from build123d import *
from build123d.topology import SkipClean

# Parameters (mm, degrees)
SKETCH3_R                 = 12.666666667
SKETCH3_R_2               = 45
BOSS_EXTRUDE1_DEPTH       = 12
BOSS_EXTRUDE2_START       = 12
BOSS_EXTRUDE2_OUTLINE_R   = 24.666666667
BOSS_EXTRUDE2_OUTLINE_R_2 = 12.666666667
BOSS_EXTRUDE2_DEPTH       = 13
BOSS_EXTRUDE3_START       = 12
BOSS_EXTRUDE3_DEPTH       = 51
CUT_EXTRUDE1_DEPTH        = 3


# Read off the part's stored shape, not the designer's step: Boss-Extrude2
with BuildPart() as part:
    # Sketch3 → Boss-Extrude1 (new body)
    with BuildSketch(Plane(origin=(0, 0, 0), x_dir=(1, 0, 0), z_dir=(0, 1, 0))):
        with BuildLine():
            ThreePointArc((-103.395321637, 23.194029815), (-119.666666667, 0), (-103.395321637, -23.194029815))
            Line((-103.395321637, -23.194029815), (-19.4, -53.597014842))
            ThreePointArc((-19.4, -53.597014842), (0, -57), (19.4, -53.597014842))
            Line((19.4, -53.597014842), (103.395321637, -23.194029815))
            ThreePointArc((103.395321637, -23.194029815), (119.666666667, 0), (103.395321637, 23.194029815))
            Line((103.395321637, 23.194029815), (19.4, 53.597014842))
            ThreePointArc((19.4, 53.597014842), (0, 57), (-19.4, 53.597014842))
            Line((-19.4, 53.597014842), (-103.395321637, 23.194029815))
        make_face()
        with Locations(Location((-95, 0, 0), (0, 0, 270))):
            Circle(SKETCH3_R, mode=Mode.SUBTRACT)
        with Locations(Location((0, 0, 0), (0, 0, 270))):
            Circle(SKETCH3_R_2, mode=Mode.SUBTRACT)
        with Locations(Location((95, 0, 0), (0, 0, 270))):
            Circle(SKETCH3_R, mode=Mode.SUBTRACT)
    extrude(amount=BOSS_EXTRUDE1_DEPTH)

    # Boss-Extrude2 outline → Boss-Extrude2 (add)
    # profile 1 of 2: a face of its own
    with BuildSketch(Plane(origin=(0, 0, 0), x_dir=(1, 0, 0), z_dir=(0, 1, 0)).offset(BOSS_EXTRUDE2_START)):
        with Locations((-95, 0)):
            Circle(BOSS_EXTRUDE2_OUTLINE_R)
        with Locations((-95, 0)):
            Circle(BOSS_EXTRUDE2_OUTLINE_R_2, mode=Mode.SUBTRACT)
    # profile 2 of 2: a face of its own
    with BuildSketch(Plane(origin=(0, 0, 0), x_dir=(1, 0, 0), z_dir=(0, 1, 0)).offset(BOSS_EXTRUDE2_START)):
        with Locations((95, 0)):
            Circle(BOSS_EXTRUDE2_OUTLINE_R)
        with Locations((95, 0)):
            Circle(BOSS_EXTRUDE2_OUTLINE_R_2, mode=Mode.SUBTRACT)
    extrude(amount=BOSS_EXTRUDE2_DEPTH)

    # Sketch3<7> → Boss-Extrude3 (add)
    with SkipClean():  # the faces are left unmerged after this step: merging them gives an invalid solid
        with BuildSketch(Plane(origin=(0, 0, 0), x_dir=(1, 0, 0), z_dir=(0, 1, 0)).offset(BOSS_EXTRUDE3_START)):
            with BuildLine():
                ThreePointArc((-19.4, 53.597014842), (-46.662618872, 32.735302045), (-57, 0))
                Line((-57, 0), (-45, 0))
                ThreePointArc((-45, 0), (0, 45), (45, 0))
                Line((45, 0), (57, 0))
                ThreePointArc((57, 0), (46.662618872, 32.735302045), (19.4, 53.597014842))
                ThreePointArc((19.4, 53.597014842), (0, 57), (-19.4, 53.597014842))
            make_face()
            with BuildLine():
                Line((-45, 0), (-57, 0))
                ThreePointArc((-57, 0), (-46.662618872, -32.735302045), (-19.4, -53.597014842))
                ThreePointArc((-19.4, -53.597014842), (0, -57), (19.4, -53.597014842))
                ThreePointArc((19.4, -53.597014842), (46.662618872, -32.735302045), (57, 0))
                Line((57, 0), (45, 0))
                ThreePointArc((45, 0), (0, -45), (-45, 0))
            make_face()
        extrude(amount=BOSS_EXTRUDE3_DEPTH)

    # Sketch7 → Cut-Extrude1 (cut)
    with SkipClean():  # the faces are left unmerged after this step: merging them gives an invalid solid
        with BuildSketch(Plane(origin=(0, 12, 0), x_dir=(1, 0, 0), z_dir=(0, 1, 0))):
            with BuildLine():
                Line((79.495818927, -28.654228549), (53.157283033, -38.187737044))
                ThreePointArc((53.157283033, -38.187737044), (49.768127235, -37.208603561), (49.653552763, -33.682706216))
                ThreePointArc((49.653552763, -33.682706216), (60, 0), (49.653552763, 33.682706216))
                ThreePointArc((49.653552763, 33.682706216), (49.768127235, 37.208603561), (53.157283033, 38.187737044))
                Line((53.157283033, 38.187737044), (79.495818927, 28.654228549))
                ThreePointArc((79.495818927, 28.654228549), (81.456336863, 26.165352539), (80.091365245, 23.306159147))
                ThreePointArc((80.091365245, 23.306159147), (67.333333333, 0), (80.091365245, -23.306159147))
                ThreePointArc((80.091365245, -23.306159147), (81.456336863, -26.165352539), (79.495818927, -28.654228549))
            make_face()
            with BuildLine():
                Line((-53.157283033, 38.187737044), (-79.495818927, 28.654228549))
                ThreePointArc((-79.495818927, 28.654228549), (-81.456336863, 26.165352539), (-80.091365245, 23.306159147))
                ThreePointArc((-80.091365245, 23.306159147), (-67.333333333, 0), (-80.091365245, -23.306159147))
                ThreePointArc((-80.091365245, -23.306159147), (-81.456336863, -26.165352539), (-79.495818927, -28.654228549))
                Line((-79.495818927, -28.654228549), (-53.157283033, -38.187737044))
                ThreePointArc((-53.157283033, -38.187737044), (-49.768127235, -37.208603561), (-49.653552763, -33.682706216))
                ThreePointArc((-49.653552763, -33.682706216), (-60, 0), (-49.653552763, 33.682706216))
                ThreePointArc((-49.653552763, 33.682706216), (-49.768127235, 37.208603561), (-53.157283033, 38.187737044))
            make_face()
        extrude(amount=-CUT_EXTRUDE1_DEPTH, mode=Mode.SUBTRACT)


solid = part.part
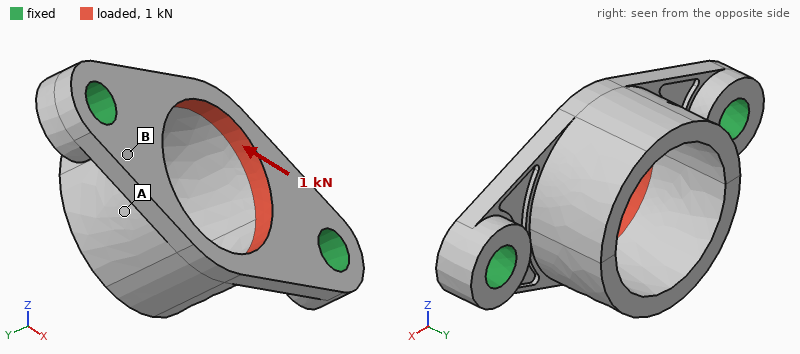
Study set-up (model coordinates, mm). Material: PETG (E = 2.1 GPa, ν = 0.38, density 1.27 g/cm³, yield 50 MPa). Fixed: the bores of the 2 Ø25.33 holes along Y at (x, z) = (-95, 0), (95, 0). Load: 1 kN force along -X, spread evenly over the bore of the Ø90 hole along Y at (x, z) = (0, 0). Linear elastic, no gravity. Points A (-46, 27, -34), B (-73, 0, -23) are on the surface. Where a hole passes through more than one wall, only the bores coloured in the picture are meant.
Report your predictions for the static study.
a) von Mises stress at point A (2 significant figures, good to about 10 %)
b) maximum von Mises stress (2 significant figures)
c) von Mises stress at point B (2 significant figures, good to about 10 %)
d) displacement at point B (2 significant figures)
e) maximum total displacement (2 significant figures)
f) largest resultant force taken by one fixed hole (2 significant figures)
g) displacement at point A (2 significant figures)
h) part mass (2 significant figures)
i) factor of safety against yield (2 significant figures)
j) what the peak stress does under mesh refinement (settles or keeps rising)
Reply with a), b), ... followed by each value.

a) 0.23 MPa
b) 1.6 MPa
c) 0.61 MPa
d) 11 µm
e) 43 µm
f) 500 N
g) 27 µm
h) 450 g
i) 31
j) settles
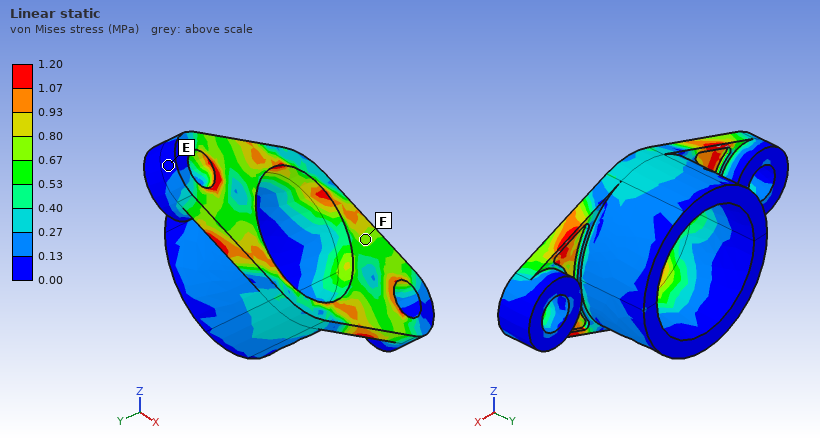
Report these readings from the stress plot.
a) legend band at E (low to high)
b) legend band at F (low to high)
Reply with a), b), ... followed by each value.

a) 0.00 to 0.13 MPa
b) 0.67 to 0.80 MPa
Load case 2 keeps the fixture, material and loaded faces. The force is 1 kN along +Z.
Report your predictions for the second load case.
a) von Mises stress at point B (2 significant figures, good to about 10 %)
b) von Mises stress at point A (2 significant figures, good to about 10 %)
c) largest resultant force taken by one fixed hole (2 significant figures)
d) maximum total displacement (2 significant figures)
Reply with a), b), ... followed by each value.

a) 1.0 MPa
b) 0.33 MPa
c) 500 N
d) 87 µm
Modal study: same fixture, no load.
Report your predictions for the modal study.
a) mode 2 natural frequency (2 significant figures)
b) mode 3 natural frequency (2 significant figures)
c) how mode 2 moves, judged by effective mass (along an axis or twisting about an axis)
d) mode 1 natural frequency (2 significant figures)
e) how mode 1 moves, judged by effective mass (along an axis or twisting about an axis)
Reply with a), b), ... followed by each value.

a) 570 Hz
b) 940 Hz
c) along Y
d) 280 Hz
e) along Z
